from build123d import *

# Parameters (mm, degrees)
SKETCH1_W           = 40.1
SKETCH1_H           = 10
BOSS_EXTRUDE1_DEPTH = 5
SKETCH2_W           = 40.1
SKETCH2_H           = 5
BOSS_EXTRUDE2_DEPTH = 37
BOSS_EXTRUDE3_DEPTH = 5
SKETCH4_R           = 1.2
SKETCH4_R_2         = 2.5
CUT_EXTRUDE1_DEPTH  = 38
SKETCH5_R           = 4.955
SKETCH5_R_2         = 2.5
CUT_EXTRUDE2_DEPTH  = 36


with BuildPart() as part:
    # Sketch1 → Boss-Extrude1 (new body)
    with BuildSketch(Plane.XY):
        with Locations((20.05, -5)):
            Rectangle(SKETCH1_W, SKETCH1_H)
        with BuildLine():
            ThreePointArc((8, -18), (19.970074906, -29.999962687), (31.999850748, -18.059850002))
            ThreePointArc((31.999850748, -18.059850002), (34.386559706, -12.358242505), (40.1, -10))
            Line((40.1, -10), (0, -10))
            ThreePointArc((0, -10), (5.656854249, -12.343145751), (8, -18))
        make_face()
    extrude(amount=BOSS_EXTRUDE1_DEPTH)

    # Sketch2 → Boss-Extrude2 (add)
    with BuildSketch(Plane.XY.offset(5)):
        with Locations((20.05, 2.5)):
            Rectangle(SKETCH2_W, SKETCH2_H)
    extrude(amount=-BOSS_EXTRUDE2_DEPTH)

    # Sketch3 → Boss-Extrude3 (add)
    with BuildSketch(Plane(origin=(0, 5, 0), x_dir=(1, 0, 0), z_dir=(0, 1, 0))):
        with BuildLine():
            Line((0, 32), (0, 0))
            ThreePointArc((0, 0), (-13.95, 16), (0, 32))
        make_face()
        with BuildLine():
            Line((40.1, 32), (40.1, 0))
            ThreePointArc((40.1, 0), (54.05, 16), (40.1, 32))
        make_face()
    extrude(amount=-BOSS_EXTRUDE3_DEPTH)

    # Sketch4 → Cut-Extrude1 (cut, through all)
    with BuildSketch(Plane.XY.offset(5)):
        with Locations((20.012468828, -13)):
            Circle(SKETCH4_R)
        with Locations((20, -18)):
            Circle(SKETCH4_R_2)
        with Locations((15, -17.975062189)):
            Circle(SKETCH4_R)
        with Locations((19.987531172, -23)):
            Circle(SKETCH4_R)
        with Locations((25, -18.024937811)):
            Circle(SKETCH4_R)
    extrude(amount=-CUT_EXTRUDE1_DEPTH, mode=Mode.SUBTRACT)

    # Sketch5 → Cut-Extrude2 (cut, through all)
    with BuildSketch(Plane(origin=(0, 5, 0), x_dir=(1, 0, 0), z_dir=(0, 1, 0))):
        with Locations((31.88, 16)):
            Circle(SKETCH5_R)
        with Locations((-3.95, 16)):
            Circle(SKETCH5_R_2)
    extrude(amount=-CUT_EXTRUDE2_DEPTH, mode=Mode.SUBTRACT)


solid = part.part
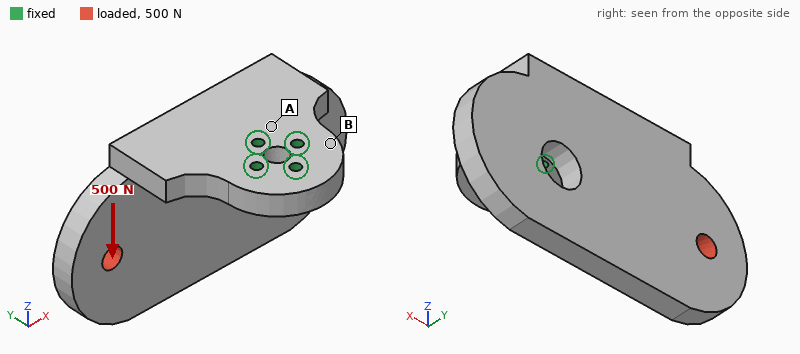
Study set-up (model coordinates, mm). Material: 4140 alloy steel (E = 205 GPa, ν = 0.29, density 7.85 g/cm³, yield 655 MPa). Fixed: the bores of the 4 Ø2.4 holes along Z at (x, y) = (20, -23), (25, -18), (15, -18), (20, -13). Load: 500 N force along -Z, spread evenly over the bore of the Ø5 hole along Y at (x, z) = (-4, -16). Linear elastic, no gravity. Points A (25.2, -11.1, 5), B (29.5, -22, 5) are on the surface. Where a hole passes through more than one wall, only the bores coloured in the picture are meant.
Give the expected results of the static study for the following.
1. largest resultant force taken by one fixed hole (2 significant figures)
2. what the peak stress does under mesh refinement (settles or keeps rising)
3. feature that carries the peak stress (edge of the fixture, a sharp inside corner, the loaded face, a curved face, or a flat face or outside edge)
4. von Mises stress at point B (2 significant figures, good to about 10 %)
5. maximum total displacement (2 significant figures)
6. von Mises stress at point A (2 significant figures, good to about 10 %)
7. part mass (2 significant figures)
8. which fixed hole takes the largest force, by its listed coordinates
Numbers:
770 N
keeps rising
edge of the fixture
22 MPa
92 µm
69 MPa
110 g
(20, -13)
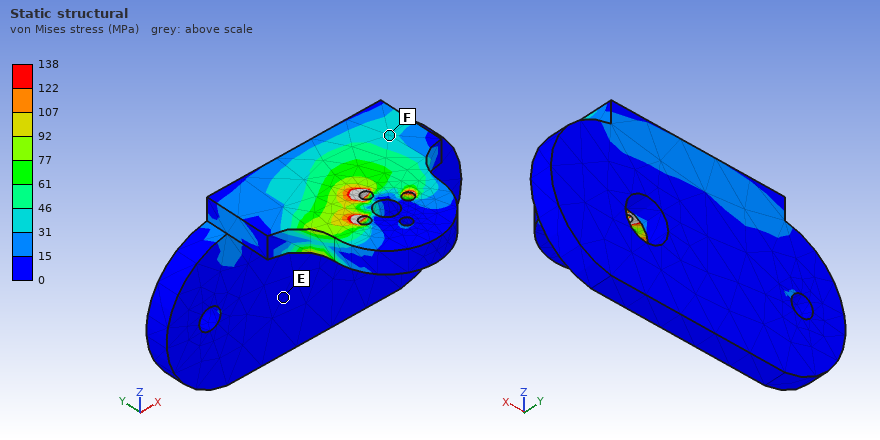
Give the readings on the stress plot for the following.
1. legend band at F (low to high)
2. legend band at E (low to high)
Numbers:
31 to 46 MPa
0 to 15 MPa
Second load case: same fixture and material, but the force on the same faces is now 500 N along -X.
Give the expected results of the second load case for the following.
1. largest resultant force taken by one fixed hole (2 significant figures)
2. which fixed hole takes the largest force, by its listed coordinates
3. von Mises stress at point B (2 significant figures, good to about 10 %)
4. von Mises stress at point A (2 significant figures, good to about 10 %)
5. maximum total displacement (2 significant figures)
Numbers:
690 N
(20, -13)
27 MPa
41 MPa
53 µm
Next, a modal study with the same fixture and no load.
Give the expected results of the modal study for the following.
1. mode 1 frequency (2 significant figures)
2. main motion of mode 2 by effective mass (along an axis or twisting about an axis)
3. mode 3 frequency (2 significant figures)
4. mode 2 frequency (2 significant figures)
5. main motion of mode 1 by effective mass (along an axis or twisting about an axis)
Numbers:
1500 Hz
along X
3600 Hz
1800 Hz
along Y
